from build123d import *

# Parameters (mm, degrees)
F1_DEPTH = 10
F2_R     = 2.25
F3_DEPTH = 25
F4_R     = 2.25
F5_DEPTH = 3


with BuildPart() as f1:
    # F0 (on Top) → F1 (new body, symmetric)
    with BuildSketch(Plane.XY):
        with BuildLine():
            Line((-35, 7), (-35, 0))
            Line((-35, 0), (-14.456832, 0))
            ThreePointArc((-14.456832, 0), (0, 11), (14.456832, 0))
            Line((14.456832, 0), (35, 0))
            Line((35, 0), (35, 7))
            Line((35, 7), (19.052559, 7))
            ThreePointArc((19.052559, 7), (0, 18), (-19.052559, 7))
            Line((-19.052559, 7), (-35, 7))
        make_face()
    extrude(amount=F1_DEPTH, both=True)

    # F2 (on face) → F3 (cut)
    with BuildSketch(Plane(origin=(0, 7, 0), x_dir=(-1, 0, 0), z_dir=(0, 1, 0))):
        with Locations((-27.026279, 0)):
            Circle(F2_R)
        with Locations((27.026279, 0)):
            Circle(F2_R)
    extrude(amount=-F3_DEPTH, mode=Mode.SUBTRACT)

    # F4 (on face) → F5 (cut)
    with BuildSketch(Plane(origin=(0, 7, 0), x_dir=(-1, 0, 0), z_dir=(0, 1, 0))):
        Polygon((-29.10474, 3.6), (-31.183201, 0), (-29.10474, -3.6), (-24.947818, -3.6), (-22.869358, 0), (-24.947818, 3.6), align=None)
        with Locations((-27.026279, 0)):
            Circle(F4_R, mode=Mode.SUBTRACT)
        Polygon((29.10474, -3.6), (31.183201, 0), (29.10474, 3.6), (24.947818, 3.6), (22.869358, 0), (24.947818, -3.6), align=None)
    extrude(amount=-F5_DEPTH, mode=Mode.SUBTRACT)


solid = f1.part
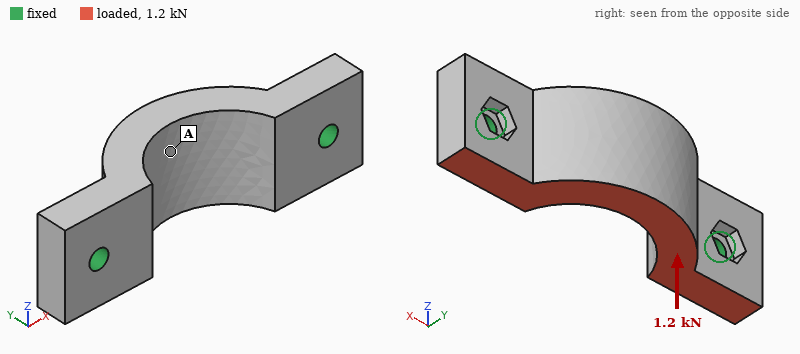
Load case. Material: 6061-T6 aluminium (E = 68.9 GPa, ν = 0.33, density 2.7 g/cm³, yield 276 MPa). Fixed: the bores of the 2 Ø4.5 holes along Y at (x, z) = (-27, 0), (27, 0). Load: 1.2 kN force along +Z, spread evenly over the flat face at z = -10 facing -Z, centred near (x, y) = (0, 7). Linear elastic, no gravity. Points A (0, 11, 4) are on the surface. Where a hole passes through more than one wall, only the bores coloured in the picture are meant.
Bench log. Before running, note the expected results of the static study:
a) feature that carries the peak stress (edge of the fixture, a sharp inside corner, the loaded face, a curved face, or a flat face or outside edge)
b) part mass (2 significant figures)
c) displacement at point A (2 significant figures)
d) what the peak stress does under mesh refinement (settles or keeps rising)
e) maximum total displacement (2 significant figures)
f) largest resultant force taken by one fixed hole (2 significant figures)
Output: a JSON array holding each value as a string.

["edge of the fixture", "29 g", "19 µm", "keeps rising", "32 µm", "600 N"]
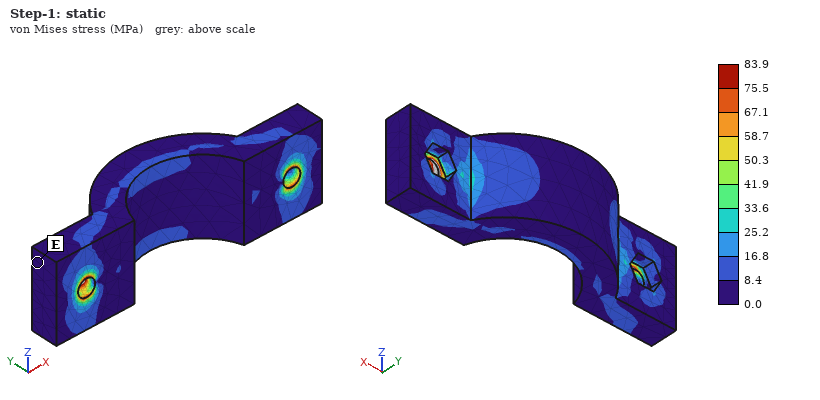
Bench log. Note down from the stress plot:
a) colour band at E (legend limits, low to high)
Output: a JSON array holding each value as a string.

["0.0 to 8.4 MPa"]
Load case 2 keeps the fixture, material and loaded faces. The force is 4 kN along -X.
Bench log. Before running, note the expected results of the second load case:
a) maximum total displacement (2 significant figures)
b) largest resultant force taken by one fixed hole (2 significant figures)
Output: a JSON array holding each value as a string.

["20 µm", "2.1 kN"]
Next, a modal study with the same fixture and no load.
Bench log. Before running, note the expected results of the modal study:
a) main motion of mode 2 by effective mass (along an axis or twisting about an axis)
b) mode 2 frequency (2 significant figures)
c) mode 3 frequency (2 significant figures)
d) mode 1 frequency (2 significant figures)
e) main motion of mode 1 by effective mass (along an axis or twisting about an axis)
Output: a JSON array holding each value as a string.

["along Y", "14 kHz", "18 kHz", "6700 Hz", "along Z"]
